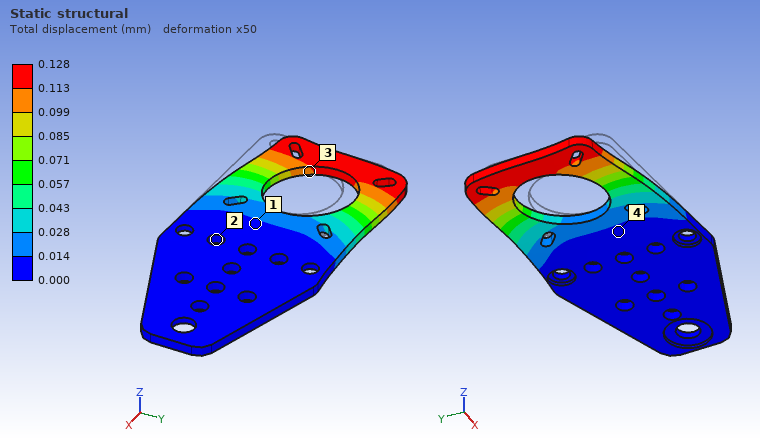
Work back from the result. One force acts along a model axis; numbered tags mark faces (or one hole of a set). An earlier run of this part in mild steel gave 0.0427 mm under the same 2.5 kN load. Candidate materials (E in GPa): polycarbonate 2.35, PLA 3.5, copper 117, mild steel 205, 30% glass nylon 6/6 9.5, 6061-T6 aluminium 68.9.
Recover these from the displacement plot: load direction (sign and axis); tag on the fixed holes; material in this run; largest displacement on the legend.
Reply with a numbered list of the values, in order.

1. +Y
2. 2
3. 6061-T6 aluminium
4. 0.128 mm
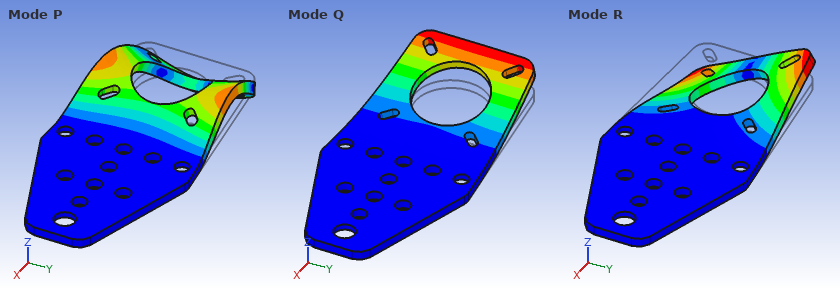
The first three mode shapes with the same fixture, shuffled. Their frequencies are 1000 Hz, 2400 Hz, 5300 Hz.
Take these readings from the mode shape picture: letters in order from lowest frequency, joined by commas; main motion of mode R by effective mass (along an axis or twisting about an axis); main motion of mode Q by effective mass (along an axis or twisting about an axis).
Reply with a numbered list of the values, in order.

1. Q, R, P
2. twisting about X
3. along Z
